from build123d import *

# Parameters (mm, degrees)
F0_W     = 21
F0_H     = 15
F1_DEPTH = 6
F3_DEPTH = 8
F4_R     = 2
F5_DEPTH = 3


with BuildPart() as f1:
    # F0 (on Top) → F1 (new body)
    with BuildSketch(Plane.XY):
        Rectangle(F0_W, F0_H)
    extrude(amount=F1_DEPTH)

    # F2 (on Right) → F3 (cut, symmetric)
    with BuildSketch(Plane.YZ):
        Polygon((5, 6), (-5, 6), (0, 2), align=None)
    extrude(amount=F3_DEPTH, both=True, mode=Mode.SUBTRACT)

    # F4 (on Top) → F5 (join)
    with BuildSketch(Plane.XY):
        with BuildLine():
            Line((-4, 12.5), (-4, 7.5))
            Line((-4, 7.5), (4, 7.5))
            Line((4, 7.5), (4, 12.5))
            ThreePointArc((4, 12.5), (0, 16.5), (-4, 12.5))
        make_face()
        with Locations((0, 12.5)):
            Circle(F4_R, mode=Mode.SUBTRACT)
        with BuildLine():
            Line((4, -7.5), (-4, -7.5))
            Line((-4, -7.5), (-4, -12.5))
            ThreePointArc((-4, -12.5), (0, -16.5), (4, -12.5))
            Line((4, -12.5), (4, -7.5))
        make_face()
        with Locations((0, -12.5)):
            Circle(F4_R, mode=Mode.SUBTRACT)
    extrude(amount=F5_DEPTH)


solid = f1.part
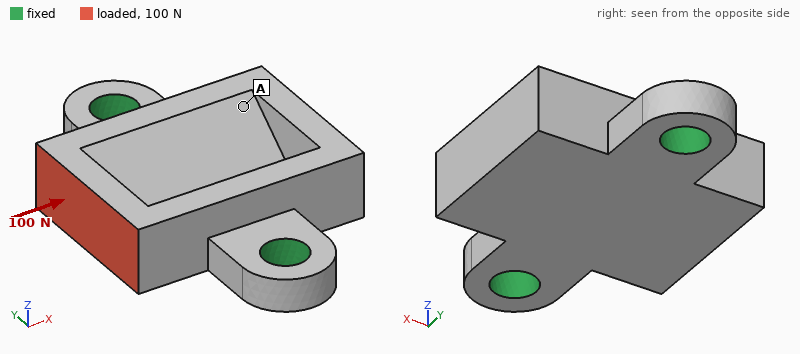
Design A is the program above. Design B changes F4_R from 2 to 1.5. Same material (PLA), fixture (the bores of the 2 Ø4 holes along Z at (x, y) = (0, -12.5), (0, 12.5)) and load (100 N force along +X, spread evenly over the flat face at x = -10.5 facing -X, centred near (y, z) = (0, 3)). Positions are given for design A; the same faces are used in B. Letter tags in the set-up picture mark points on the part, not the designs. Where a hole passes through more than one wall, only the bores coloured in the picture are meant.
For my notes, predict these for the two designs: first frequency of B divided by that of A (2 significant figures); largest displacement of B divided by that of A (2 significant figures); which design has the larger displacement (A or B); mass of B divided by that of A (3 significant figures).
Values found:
0.91
1.2
B
1.02
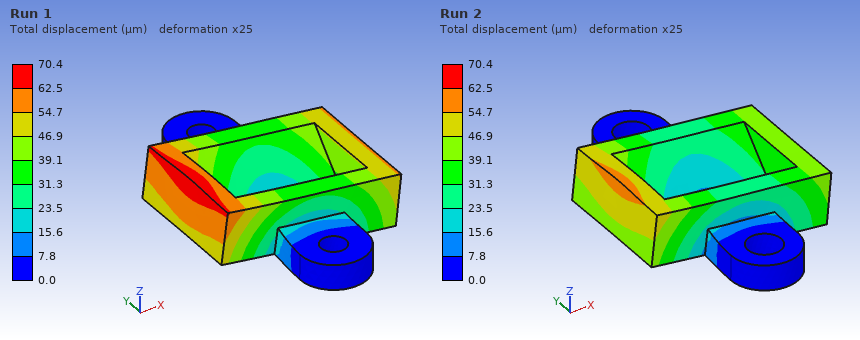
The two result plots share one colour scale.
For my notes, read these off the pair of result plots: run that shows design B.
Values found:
Run 1
